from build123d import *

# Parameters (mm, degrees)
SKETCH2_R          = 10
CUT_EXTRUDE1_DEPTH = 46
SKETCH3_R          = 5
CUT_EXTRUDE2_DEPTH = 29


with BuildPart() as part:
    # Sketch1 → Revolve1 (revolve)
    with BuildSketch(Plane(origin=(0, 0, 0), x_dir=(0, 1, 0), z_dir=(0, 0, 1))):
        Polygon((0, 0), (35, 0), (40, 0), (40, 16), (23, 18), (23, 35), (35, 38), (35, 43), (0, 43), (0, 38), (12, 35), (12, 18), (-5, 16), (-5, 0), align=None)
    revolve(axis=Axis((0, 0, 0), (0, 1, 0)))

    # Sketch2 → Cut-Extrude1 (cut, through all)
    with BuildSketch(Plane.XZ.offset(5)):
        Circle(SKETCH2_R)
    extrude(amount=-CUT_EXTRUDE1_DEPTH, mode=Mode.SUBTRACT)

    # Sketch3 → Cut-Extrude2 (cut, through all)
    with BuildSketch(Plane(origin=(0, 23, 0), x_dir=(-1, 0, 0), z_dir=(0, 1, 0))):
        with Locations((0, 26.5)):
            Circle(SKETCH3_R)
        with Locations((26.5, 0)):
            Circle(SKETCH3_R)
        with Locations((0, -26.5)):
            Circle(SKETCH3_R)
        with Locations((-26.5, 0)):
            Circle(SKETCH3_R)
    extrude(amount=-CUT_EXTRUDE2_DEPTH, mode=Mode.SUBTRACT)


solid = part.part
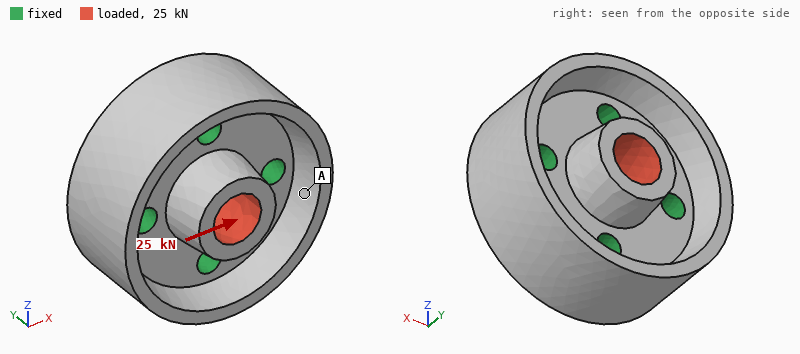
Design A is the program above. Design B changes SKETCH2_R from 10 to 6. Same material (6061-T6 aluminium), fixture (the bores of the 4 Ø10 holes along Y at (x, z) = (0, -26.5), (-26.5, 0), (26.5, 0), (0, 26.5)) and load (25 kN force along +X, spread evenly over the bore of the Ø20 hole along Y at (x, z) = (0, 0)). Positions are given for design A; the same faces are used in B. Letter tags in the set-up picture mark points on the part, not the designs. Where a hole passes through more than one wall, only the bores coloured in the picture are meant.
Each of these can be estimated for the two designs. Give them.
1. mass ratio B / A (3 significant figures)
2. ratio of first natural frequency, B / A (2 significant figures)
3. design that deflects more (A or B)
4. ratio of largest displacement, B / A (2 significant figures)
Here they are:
1.08
1.0
A
0.78
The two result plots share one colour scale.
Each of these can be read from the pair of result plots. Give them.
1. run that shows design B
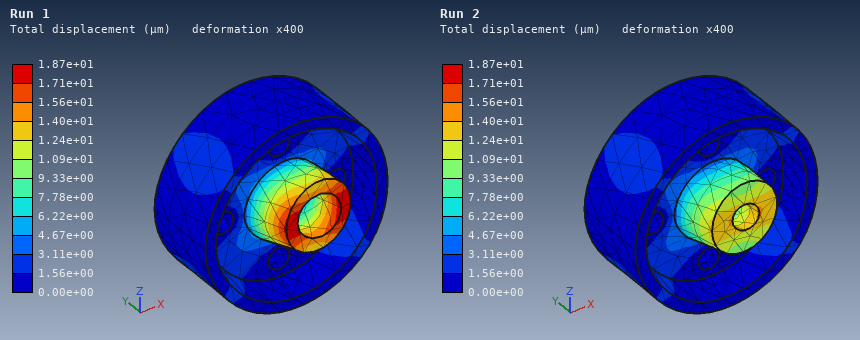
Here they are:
Run 2
